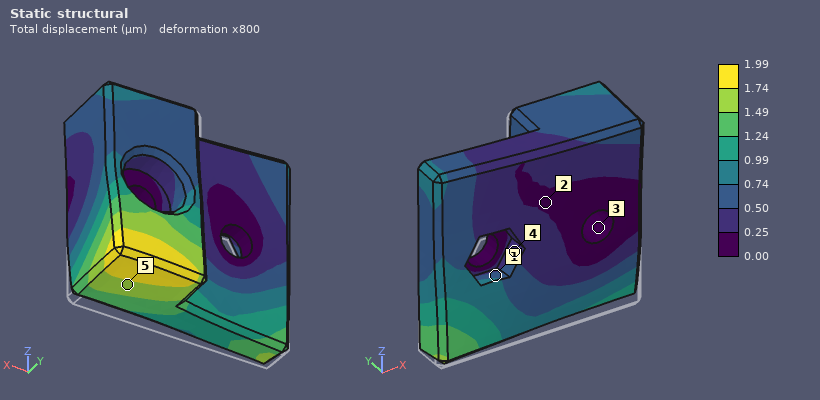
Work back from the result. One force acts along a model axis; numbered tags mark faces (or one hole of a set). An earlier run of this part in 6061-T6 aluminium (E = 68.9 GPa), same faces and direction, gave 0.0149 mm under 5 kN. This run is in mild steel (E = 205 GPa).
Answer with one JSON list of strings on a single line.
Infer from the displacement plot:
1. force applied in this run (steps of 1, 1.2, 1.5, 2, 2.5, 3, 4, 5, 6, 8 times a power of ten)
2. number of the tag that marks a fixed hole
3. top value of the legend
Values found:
["2 kN", "3", "1.99 µm"]
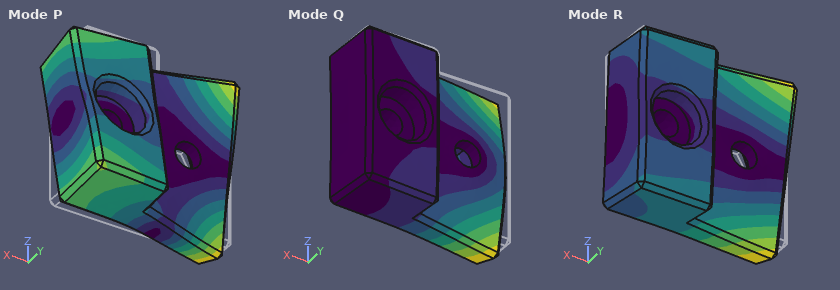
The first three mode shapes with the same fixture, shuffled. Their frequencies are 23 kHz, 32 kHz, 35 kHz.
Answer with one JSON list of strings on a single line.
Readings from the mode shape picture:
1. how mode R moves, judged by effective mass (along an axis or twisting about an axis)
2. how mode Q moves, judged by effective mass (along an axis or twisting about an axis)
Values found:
["twisting about X", "along Y"]
